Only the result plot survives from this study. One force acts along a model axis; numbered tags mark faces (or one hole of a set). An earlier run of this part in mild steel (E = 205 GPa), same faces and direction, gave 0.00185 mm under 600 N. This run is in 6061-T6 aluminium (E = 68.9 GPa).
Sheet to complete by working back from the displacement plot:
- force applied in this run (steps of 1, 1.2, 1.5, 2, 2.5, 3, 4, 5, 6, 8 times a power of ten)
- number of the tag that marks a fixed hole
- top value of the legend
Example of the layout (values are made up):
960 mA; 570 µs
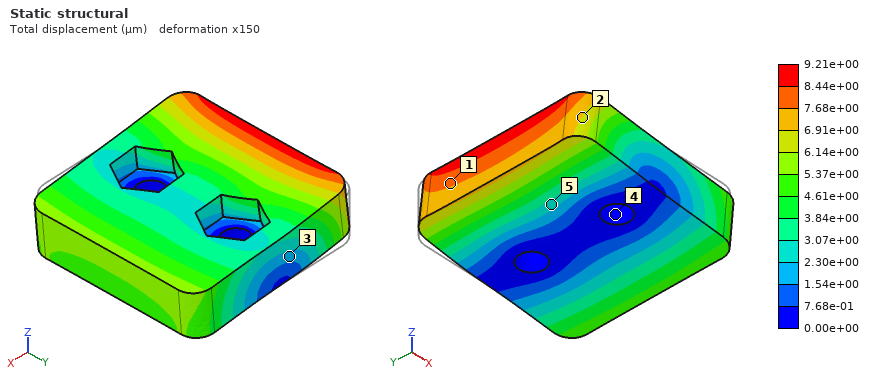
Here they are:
1 kN; 4; 9.21e+00 µm
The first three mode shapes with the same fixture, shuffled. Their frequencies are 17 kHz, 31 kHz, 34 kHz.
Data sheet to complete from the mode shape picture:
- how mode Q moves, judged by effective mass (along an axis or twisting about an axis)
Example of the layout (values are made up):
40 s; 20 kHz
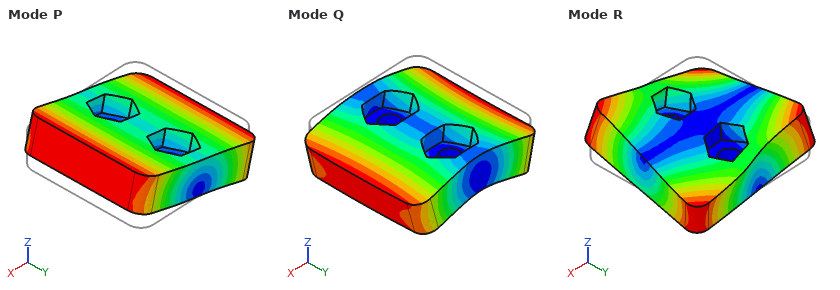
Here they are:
along Z
